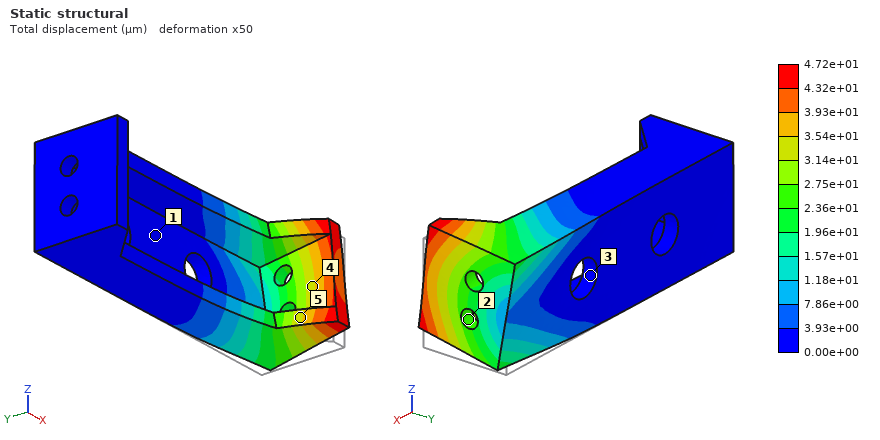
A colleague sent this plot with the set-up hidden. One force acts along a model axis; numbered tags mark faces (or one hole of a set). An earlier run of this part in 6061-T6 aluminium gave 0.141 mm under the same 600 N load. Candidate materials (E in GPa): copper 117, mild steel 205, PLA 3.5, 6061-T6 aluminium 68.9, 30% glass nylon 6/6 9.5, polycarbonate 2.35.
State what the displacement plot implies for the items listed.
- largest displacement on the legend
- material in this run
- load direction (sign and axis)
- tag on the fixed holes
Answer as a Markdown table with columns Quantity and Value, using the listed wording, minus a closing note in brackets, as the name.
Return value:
| Quantity | Value |
|---|---|
| largest displacement on the legend | 4.72e+01 µm |
| material in this run | mild steel |
| load direction | +Z |
| tag on the fixed holes | 3 |
